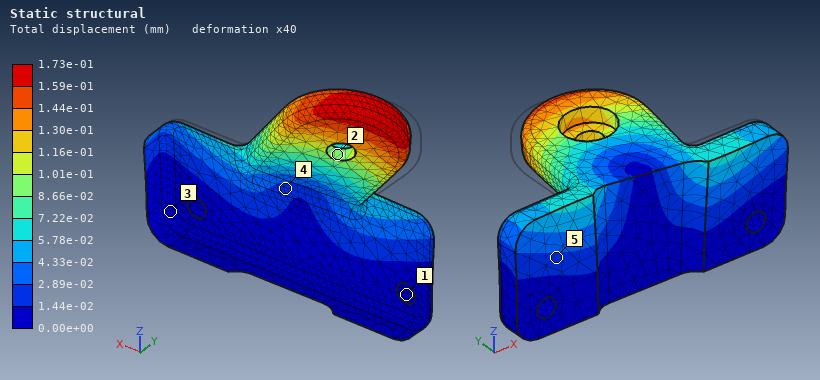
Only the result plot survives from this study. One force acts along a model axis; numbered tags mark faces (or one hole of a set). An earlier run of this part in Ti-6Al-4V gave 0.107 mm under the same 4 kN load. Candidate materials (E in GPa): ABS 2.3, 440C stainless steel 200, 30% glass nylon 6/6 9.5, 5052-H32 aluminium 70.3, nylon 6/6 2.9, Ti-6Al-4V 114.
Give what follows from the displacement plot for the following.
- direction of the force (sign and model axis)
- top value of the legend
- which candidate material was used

+X
1.73e-01 mm
5052-H32 aluminium
